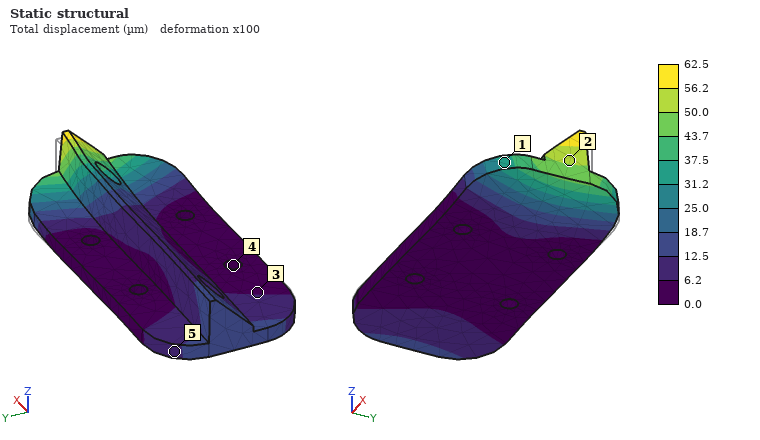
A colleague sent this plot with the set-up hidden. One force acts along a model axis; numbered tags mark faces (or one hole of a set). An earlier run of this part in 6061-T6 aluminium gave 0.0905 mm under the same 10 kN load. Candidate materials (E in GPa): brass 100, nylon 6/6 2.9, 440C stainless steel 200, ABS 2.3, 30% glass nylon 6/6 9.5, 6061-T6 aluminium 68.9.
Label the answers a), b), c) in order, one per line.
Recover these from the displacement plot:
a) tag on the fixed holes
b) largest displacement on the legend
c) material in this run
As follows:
a) 4
b) 62.5 µm
c) brass
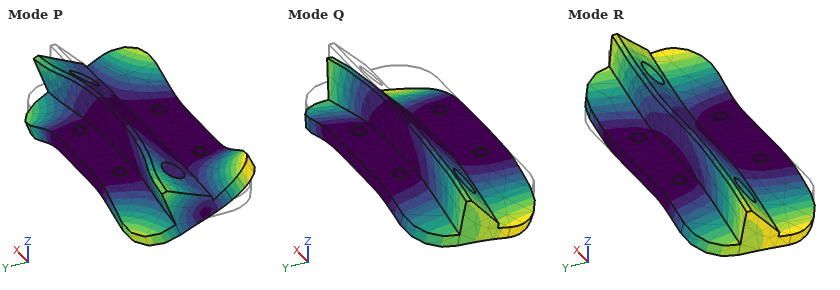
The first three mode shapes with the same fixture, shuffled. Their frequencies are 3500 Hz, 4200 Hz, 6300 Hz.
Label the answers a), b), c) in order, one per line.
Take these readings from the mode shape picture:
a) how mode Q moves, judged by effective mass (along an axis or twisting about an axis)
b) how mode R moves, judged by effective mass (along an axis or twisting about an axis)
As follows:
a) along Z
b) twisting about Y
